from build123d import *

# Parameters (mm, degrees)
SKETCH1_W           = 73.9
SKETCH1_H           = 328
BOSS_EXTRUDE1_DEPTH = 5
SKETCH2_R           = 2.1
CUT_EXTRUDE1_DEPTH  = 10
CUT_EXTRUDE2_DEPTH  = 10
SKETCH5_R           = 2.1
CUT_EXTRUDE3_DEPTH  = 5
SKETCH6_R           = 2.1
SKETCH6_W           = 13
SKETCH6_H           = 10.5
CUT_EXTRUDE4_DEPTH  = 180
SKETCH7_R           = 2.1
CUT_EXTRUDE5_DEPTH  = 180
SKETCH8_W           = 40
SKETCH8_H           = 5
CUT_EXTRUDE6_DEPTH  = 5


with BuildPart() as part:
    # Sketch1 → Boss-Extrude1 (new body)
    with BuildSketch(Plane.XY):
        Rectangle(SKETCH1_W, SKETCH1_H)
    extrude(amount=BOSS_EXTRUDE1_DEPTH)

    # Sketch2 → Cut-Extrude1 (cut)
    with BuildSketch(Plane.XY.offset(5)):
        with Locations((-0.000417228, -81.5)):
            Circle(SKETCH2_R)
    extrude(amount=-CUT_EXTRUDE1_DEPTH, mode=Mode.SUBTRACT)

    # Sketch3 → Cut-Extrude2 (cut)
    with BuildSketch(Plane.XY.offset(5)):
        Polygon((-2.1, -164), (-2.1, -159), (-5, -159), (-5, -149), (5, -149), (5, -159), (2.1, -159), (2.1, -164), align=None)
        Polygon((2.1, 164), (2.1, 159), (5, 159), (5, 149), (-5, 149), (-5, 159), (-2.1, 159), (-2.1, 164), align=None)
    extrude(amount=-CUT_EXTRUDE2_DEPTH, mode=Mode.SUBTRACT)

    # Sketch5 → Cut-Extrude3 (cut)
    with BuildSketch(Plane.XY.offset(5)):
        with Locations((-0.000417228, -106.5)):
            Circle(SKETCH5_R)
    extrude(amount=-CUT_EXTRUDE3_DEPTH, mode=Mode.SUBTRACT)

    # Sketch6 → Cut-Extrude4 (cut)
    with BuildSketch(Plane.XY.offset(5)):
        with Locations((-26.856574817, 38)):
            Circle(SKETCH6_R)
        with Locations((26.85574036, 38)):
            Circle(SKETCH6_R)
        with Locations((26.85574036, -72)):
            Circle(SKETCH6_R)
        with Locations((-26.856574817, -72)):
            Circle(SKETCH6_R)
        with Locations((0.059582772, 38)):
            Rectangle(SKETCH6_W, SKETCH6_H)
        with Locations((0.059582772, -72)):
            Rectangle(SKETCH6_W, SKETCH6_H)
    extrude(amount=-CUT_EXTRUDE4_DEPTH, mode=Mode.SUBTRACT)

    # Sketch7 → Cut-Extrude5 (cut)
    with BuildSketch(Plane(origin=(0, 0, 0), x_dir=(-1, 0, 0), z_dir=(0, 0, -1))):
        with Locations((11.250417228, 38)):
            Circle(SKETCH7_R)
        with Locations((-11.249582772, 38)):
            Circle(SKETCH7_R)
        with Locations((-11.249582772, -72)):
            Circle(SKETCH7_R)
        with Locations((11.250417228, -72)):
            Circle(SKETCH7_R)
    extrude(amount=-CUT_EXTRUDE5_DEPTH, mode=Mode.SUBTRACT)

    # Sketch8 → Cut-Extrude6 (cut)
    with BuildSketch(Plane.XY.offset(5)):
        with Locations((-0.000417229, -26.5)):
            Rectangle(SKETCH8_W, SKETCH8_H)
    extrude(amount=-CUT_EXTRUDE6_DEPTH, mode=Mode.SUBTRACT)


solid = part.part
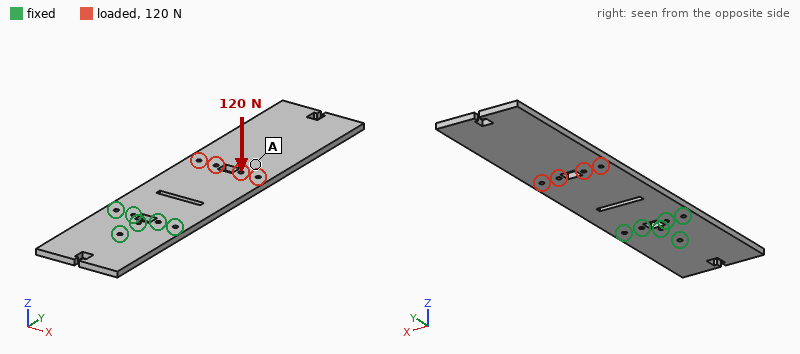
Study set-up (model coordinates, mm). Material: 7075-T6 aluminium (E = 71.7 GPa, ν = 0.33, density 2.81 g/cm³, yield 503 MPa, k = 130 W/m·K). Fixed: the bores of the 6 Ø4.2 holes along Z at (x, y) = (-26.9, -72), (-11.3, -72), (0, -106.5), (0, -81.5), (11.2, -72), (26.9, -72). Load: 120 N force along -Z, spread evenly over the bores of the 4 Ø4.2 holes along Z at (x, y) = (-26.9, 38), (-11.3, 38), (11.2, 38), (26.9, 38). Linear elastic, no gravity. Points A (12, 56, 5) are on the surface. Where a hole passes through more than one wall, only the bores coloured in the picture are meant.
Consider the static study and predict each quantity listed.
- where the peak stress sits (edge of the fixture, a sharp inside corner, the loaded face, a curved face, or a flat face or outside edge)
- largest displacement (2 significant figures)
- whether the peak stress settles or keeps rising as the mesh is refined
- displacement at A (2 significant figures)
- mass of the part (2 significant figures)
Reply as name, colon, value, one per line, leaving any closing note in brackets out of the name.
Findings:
where the peak stress sits: edge of the fixture
largest displacement: 3.3 mm
whether the peak stress settles or keeps rising as the mesh is refined: keeps rising
displacement at A: 1.5 mm
mass of the part: 330 g
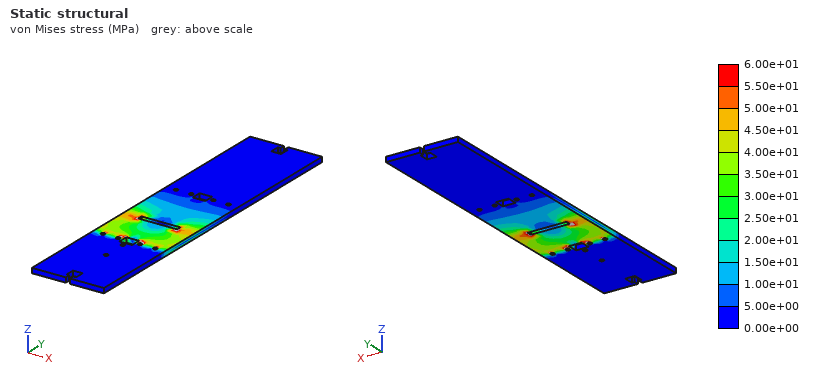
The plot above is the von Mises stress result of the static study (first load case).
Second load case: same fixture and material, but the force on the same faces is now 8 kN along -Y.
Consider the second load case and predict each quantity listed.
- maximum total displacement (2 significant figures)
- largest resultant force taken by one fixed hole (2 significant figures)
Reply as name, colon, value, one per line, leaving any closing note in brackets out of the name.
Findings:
maximum total displacement: 53 µm
largest resultant force taken by one fixed hole: 2.3 kN
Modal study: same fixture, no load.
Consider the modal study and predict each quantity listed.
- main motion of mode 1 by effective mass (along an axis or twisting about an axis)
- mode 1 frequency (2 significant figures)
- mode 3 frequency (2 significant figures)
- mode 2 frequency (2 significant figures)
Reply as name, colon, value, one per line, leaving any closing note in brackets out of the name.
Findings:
main motion of mode 1 by effective mass: along Z
mode 1 frequency: 67 Hz
mode 3 frequency: 460 Hz
mode 2 frequency: 450 Hz
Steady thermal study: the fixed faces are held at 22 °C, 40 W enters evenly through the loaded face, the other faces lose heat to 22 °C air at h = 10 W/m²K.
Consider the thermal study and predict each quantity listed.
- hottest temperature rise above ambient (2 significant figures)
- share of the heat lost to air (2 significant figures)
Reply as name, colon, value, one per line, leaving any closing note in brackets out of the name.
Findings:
hottest temperature rise above ambient: 72 K
share of the heat lost to air: 45 %
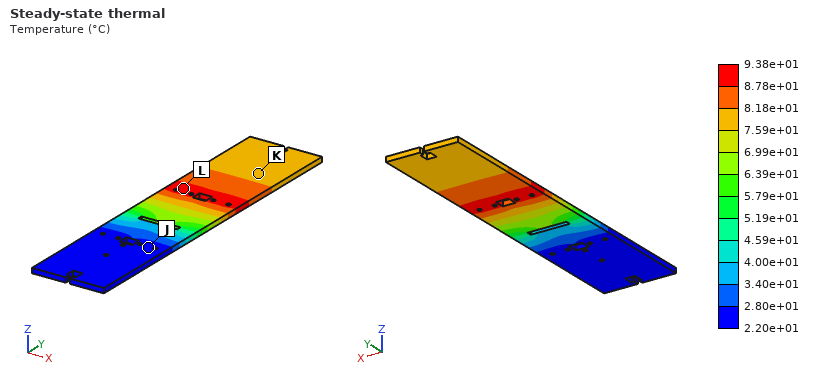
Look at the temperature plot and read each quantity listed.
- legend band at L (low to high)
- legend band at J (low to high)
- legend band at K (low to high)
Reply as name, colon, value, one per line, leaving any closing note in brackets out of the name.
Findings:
legend band at L: 8.78e+01 to 9.38e+01 °C
legend band at J: 2.20e+01 to 2.80e+01 °C
legend band at K: 7.59e+01 to 8.18e+01 °C
